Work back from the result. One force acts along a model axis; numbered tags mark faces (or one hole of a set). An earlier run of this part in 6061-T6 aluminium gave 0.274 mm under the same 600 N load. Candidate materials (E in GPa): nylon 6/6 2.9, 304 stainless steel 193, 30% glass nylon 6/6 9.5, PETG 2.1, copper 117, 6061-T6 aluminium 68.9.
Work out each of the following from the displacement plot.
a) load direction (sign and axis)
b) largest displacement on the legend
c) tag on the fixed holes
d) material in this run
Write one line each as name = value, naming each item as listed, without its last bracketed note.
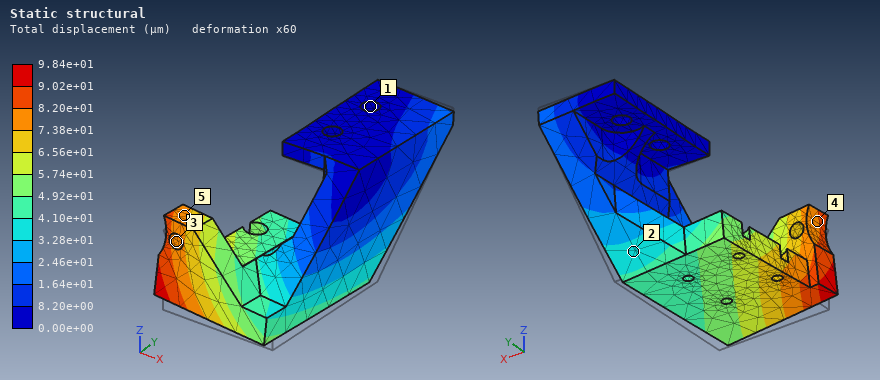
load direction = +Z
largest displacement on the legend = 9.84e+01 µm
tag on the fixed holes = 1
material in this run = 304 stainless steel
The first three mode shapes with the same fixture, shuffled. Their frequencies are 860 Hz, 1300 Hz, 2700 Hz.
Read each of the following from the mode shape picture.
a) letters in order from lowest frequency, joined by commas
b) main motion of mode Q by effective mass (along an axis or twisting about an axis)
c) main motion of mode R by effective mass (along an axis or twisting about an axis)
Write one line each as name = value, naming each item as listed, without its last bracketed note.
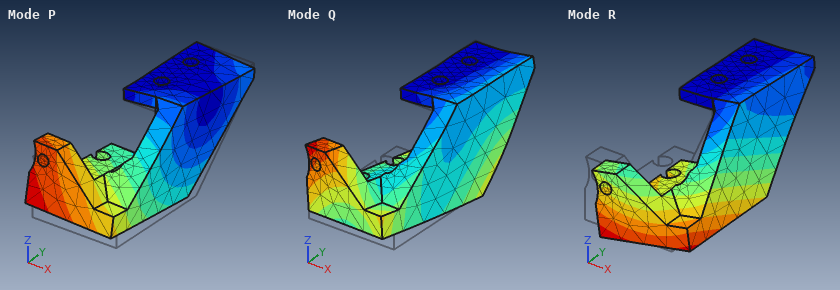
letters in order from lowest frequency, joined by commas = R, P, Q
main motion of mode Q by effective mass = along Z
main motion of mode R by effective mass = along X
